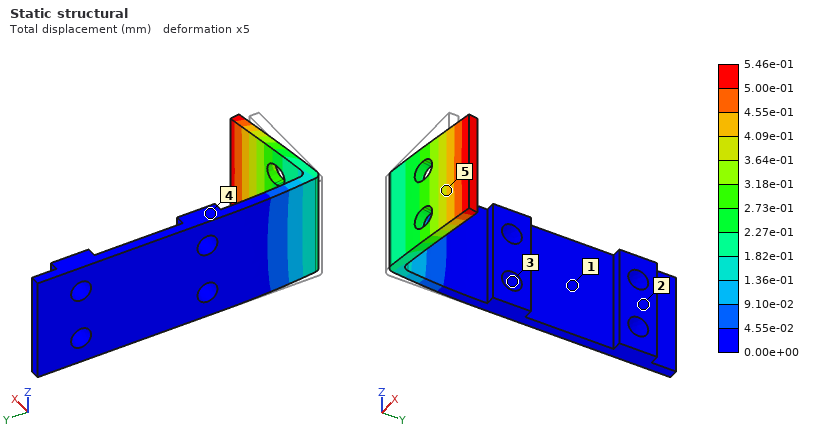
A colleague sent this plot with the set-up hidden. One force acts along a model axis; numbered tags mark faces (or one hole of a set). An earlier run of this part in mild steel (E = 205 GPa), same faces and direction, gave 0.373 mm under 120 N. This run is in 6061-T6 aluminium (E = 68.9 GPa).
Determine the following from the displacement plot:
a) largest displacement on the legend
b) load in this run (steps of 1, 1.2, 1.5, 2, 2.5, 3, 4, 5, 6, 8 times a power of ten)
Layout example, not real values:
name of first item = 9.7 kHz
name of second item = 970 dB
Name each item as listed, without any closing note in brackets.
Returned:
largest displacement on the legend = 5.46e-01 mm
load in this run = 60 N
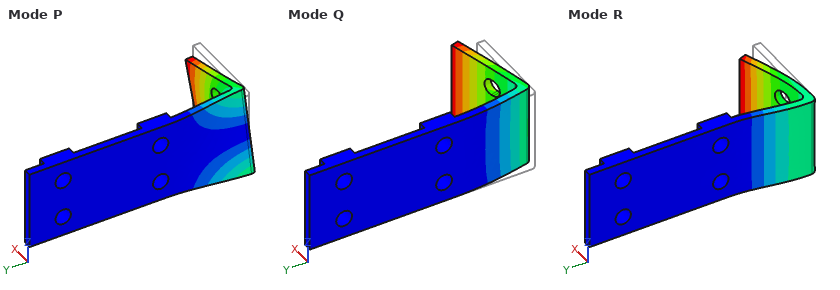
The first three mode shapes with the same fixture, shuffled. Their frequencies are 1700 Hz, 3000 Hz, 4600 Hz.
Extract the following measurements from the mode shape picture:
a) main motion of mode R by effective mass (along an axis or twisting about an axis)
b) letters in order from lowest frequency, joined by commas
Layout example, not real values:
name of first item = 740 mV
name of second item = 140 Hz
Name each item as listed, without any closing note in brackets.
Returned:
main motion of mode R by effective mass = along X
letters in order from lowest frequency, joined by commas = Q, P, R
